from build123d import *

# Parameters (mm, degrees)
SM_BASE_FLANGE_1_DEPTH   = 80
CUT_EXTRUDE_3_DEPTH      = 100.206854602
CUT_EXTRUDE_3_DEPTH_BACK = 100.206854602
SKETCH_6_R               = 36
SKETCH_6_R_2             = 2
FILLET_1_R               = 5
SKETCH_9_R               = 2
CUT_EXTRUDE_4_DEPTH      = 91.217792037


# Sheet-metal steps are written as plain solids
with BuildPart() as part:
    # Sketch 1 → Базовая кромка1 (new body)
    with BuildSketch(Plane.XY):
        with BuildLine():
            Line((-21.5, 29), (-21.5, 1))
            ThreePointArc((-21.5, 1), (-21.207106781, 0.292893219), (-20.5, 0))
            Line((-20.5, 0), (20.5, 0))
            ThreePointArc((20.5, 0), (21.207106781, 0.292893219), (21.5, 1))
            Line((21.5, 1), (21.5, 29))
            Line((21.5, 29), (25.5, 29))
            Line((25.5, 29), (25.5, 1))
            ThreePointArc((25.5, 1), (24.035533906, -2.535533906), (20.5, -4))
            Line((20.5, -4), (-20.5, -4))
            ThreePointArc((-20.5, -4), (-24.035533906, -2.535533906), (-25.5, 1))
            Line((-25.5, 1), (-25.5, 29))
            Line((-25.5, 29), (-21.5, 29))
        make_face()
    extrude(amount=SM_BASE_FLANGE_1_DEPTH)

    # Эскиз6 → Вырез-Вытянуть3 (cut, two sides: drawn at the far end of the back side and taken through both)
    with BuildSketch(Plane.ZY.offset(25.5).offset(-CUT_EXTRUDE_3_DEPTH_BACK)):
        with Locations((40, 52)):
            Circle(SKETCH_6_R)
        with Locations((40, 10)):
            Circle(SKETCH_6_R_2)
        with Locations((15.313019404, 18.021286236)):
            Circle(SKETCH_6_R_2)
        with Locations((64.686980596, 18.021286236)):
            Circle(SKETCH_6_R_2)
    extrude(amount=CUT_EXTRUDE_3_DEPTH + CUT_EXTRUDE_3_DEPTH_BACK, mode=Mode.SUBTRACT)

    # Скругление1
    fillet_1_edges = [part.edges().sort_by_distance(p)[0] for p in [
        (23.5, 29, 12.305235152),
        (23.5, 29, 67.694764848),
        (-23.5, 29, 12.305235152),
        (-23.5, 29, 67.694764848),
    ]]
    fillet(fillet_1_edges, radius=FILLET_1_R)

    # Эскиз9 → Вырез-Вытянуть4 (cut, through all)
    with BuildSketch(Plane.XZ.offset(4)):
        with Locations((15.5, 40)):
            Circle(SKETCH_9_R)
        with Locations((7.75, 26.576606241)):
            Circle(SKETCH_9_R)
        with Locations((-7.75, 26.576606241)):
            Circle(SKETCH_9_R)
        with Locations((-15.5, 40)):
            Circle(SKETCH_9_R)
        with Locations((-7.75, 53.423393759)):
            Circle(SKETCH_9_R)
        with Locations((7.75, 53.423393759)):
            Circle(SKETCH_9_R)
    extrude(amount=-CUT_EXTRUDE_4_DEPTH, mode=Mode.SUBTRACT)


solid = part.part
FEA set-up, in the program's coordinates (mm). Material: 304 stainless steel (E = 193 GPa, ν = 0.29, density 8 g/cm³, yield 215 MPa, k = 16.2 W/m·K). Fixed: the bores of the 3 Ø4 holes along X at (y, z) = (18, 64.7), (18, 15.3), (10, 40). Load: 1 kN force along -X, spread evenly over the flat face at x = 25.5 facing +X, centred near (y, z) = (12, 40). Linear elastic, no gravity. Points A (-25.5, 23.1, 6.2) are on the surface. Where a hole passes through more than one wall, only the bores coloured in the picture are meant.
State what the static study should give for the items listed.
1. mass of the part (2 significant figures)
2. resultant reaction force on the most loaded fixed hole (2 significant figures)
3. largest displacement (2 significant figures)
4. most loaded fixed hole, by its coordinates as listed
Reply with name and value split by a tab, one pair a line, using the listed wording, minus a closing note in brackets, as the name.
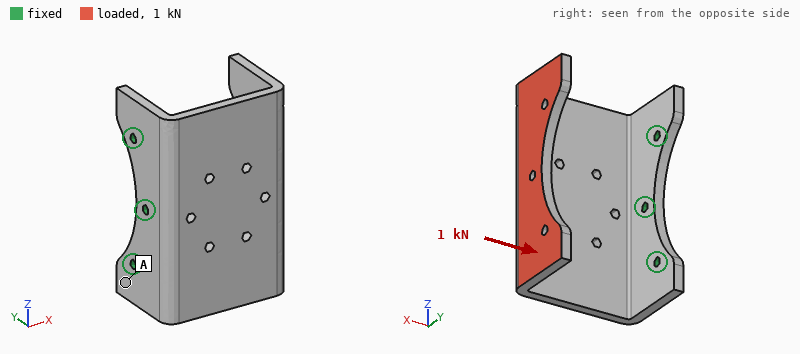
mass of the part	240 g
resultant reaction force on the most loaded fixed hole	410 N
largest displacement	0.40 mm
most loaded fixed hole, by its coordinates as listed	(10, 40)
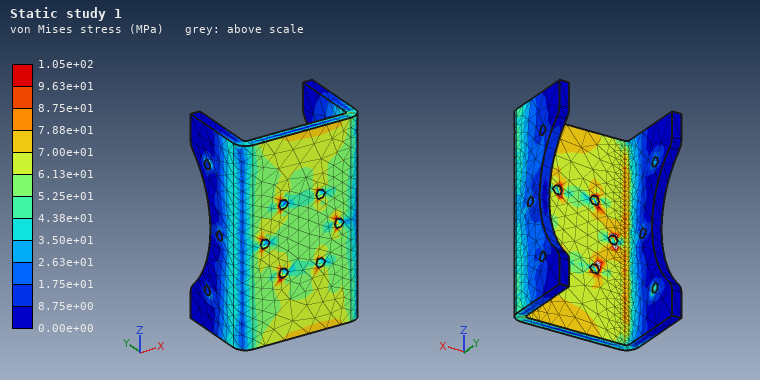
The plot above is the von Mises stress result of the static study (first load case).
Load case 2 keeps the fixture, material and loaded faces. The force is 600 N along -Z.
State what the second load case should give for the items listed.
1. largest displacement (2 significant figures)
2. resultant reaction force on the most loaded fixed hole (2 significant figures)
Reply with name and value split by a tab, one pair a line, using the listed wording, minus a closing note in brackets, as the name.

largest displacement	0.21 mm
resultant reaction force on the most loaded fixed hole	500 N
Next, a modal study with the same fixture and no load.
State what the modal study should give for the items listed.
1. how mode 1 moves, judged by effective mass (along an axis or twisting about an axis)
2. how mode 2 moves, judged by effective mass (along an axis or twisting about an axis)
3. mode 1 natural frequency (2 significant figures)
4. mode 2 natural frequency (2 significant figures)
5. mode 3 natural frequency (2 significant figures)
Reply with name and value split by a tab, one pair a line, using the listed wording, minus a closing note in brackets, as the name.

how mode 1 moves, judged by effective mass	along Y
how mode 2 moves, judged by effective mass	along Z
mode 1 natural frequency	570 Hz
mode 2 natural frequency	990 Hz
mode 3 natural frequency	1800 Hz
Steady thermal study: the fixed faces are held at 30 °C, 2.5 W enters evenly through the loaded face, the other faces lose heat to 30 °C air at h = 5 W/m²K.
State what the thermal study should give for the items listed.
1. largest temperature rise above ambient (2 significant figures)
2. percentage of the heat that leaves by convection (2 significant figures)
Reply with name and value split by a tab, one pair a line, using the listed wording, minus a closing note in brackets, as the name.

largest temperature rise above ambient	29 K
percentage of the heat that leaves by convection	38 %
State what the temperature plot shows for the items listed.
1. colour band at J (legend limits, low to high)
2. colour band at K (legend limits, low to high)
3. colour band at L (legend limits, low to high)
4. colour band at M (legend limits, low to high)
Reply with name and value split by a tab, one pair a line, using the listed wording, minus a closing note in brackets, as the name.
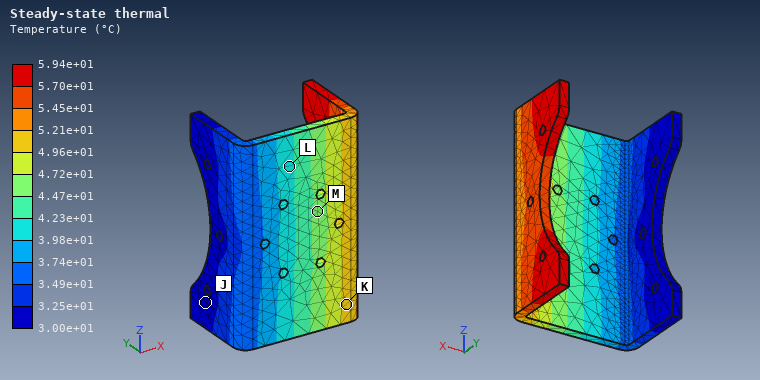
colour band at J	3.00e+01 to 3.25e+01 °C
colour band at K	4.96e+01 to 5.21e+01 °C
colour band at L	3.98e+01 to 4.23e+01 °C
colour band at M	4.47e+01 to 4.72e+01 °C
